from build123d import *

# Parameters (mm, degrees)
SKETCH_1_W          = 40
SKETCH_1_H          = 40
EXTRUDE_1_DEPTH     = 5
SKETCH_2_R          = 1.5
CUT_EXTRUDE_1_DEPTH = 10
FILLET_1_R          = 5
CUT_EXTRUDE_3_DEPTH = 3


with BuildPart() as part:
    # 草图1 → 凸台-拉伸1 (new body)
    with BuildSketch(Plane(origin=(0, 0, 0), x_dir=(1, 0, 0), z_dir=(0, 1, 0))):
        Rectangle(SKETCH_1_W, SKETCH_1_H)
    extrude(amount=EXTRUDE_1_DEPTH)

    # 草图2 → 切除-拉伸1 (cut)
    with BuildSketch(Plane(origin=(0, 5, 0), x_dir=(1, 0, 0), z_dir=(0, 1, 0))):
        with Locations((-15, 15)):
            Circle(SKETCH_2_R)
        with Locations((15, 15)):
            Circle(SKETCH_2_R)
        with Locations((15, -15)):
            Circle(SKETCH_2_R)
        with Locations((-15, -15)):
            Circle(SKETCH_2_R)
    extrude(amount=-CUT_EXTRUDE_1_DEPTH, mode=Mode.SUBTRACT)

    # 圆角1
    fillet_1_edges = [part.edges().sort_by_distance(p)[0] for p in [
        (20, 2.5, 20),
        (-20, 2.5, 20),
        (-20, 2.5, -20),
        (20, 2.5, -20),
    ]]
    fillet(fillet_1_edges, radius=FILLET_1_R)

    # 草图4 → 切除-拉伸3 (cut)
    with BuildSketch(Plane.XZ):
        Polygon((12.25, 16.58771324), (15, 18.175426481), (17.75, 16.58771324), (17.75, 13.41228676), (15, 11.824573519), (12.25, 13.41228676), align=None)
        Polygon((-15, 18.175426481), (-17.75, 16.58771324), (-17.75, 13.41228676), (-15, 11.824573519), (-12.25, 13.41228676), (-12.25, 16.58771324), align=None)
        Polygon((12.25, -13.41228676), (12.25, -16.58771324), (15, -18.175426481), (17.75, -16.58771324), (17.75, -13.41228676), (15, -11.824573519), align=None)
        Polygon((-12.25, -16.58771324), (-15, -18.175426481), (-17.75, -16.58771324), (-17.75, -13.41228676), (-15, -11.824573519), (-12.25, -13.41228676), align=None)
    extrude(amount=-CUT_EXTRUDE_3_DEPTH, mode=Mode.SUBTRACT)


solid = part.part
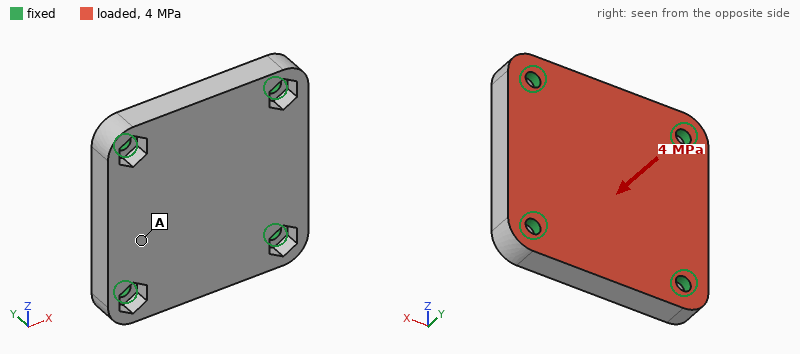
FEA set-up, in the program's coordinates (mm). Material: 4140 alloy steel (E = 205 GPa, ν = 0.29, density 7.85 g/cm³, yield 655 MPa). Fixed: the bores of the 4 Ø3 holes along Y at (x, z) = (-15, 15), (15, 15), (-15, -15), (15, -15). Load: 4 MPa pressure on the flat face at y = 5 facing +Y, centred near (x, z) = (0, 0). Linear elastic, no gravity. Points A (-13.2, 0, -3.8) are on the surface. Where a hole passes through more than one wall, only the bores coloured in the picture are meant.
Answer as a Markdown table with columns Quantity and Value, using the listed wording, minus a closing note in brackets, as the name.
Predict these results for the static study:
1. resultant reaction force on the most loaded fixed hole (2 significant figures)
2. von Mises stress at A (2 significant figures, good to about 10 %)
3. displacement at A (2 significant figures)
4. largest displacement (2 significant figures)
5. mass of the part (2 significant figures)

| Quantity | Value |
|---|---|
| resultant reaction force on the most loaded fixed hole | 1.9 kN |
| von Mises stress at A | 60 MPa |
| displacement at A | 12 µm |
| largest displacement | 18 µm |
| mass of the part | 59 g |
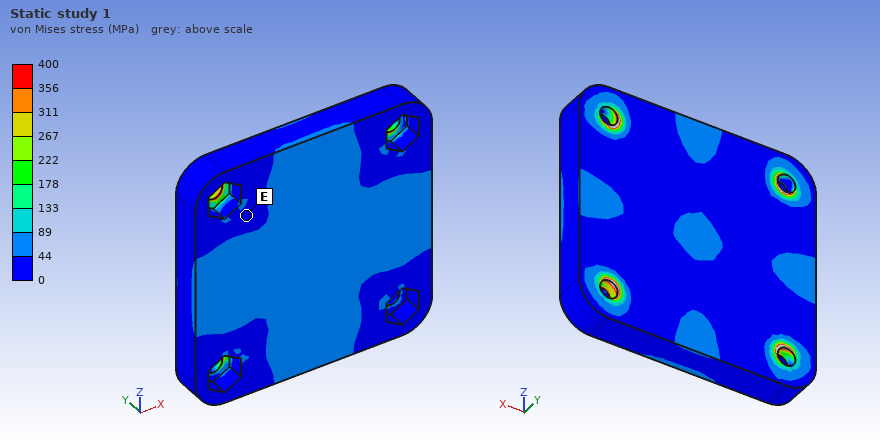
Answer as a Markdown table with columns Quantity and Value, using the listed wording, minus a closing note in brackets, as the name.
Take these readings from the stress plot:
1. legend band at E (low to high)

| Quantity | Value |
|---|---|
| legend band at E | 0 to 44 MPa |
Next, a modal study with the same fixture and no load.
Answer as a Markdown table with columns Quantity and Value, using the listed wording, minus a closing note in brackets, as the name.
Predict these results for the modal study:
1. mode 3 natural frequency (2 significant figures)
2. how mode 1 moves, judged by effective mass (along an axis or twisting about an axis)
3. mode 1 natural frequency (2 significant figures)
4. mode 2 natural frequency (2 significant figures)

| Quantity | Value |
|---|---|
| mode 3 natural frequency | 21 kHz |
| how mode 1 moves, judged by effective mass | along Y |
| mode 1 natural frequency | 14 kHz |
| mode 2 natural frequency | 21 kHz |
